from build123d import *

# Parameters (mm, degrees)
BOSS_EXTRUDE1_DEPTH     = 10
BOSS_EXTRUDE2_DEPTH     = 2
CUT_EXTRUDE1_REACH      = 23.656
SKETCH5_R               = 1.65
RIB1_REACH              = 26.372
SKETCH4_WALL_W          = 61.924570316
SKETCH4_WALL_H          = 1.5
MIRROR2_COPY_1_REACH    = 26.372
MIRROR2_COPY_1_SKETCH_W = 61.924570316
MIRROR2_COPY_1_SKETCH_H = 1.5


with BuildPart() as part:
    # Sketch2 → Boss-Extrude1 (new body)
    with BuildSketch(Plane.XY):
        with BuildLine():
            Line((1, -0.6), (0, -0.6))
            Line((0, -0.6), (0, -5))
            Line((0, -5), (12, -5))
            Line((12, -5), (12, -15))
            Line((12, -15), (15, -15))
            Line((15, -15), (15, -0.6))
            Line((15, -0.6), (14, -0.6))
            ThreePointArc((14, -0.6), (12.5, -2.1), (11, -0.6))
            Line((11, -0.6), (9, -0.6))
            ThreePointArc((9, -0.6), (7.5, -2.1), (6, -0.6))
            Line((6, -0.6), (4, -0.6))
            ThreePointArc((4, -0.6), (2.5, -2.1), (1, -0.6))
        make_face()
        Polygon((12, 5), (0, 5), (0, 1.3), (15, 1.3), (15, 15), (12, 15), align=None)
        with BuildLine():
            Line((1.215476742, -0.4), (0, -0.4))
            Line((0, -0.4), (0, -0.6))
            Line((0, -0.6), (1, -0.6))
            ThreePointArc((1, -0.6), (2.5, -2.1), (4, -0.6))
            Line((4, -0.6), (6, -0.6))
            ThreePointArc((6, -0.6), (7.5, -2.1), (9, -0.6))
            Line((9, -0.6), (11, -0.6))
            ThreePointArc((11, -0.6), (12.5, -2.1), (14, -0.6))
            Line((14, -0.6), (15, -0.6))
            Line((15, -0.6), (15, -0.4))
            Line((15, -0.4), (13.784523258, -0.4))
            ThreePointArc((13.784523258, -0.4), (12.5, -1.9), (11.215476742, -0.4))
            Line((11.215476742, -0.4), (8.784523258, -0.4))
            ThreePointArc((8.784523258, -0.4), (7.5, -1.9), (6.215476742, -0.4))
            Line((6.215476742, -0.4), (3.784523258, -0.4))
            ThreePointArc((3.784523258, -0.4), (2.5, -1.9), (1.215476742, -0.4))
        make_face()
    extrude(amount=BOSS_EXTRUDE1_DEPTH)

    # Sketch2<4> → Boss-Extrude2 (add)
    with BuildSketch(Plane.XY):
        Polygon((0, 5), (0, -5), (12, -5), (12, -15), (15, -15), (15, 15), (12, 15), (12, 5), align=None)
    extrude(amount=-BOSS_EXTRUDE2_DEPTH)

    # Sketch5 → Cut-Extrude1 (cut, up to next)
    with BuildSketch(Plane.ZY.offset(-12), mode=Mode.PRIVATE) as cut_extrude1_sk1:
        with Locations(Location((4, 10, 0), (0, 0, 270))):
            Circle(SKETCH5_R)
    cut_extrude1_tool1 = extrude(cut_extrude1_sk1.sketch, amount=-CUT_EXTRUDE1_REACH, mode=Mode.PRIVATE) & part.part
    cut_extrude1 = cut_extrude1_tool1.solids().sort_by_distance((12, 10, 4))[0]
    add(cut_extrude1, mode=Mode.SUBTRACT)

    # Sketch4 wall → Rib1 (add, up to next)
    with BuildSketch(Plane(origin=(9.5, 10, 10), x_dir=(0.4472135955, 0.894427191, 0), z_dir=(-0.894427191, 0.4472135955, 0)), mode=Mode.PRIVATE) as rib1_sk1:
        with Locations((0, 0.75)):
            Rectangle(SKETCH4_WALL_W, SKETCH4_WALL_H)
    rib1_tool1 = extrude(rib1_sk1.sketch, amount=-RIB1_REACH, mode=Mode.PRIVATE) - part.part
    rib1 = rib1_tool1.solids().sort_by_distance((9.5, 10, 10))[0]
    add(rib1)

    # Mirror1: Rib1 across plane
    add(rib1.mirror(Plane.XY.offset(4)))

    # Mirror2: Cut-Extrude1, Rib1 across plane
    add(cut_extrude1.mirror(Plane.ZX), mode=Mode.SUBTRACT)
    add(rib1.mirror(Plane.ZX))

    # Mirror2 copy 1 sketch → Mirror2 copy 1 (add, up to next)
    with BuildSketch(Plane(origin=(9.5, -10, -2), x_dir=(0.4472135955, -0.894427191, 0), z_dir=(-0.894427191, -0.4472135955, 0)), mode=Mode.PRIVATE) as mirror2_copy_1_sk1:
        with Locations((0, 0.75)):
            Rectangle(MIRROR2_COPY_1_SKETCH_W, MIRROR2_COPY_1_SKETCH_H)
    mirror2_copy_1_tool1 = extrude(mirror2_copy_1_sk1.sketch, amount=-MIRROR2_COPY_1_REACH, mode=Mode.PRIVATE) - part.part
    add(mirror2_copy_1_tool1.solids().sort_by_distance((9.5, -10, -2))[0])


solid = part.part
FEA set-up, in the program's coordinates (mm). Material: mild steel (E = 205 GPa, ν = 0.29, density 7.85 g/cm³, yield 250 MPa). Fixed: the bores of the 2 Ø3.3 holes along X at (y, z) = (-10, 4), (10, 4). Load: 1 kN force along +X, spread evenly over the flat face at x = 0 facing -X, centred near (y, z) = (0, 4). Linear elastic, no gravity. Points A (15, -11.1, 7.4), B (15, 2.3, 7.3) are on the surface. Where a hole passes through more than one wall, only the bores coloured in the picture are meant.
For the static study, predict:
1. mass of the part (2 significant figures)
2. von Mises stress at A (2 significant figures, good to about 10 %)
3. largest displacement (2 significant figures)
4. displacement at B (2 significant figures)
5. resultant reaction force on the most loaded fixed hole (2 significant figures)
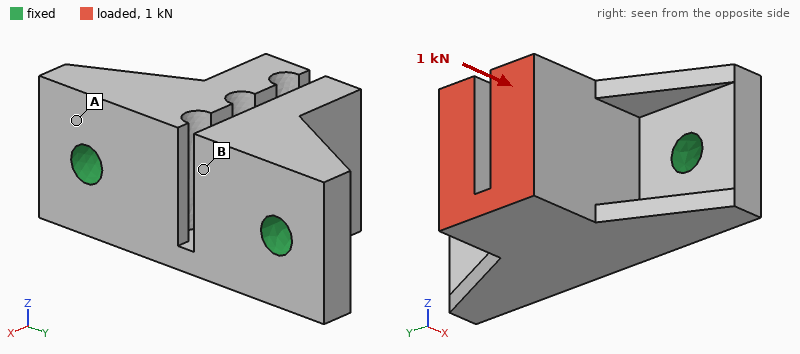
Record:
18 g
24 MPa
8.3 µm
3.7 µm
530 N
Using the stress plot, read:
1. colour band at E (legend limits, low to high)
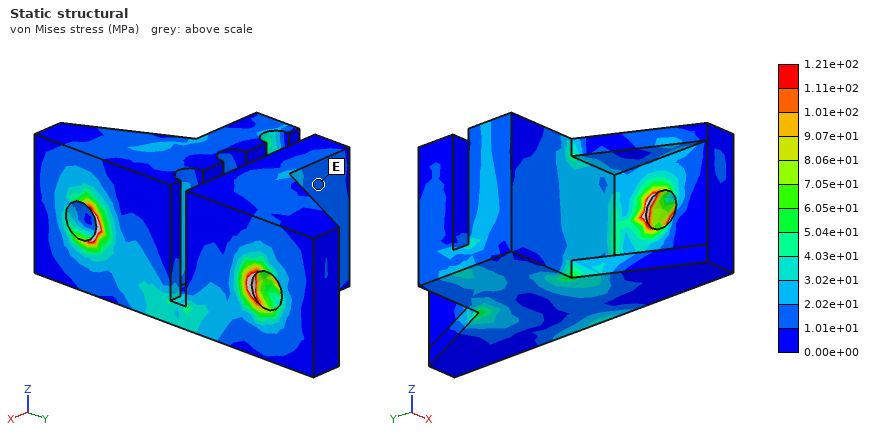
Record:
1.01e+01 to 2.02e+01 MPa
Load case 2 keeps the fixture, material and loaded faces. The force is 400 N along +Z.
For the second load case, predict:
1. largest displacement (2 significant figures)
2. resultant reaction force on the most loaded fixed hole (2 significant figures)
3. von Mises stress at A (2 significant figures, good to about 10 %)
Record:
19 µm
210 N
51 MPa
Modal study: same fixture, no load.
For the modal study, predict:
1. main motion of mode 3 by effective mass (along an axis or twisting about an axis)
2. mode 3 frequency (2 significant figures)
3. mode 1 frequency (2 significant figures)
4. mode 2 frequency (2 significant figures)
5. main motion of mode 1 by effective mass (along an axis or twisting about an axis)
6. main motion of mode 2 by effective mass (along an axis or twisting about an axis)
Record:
along X
21 kHz
12 kHz
18 kHz
along Z
along Y
